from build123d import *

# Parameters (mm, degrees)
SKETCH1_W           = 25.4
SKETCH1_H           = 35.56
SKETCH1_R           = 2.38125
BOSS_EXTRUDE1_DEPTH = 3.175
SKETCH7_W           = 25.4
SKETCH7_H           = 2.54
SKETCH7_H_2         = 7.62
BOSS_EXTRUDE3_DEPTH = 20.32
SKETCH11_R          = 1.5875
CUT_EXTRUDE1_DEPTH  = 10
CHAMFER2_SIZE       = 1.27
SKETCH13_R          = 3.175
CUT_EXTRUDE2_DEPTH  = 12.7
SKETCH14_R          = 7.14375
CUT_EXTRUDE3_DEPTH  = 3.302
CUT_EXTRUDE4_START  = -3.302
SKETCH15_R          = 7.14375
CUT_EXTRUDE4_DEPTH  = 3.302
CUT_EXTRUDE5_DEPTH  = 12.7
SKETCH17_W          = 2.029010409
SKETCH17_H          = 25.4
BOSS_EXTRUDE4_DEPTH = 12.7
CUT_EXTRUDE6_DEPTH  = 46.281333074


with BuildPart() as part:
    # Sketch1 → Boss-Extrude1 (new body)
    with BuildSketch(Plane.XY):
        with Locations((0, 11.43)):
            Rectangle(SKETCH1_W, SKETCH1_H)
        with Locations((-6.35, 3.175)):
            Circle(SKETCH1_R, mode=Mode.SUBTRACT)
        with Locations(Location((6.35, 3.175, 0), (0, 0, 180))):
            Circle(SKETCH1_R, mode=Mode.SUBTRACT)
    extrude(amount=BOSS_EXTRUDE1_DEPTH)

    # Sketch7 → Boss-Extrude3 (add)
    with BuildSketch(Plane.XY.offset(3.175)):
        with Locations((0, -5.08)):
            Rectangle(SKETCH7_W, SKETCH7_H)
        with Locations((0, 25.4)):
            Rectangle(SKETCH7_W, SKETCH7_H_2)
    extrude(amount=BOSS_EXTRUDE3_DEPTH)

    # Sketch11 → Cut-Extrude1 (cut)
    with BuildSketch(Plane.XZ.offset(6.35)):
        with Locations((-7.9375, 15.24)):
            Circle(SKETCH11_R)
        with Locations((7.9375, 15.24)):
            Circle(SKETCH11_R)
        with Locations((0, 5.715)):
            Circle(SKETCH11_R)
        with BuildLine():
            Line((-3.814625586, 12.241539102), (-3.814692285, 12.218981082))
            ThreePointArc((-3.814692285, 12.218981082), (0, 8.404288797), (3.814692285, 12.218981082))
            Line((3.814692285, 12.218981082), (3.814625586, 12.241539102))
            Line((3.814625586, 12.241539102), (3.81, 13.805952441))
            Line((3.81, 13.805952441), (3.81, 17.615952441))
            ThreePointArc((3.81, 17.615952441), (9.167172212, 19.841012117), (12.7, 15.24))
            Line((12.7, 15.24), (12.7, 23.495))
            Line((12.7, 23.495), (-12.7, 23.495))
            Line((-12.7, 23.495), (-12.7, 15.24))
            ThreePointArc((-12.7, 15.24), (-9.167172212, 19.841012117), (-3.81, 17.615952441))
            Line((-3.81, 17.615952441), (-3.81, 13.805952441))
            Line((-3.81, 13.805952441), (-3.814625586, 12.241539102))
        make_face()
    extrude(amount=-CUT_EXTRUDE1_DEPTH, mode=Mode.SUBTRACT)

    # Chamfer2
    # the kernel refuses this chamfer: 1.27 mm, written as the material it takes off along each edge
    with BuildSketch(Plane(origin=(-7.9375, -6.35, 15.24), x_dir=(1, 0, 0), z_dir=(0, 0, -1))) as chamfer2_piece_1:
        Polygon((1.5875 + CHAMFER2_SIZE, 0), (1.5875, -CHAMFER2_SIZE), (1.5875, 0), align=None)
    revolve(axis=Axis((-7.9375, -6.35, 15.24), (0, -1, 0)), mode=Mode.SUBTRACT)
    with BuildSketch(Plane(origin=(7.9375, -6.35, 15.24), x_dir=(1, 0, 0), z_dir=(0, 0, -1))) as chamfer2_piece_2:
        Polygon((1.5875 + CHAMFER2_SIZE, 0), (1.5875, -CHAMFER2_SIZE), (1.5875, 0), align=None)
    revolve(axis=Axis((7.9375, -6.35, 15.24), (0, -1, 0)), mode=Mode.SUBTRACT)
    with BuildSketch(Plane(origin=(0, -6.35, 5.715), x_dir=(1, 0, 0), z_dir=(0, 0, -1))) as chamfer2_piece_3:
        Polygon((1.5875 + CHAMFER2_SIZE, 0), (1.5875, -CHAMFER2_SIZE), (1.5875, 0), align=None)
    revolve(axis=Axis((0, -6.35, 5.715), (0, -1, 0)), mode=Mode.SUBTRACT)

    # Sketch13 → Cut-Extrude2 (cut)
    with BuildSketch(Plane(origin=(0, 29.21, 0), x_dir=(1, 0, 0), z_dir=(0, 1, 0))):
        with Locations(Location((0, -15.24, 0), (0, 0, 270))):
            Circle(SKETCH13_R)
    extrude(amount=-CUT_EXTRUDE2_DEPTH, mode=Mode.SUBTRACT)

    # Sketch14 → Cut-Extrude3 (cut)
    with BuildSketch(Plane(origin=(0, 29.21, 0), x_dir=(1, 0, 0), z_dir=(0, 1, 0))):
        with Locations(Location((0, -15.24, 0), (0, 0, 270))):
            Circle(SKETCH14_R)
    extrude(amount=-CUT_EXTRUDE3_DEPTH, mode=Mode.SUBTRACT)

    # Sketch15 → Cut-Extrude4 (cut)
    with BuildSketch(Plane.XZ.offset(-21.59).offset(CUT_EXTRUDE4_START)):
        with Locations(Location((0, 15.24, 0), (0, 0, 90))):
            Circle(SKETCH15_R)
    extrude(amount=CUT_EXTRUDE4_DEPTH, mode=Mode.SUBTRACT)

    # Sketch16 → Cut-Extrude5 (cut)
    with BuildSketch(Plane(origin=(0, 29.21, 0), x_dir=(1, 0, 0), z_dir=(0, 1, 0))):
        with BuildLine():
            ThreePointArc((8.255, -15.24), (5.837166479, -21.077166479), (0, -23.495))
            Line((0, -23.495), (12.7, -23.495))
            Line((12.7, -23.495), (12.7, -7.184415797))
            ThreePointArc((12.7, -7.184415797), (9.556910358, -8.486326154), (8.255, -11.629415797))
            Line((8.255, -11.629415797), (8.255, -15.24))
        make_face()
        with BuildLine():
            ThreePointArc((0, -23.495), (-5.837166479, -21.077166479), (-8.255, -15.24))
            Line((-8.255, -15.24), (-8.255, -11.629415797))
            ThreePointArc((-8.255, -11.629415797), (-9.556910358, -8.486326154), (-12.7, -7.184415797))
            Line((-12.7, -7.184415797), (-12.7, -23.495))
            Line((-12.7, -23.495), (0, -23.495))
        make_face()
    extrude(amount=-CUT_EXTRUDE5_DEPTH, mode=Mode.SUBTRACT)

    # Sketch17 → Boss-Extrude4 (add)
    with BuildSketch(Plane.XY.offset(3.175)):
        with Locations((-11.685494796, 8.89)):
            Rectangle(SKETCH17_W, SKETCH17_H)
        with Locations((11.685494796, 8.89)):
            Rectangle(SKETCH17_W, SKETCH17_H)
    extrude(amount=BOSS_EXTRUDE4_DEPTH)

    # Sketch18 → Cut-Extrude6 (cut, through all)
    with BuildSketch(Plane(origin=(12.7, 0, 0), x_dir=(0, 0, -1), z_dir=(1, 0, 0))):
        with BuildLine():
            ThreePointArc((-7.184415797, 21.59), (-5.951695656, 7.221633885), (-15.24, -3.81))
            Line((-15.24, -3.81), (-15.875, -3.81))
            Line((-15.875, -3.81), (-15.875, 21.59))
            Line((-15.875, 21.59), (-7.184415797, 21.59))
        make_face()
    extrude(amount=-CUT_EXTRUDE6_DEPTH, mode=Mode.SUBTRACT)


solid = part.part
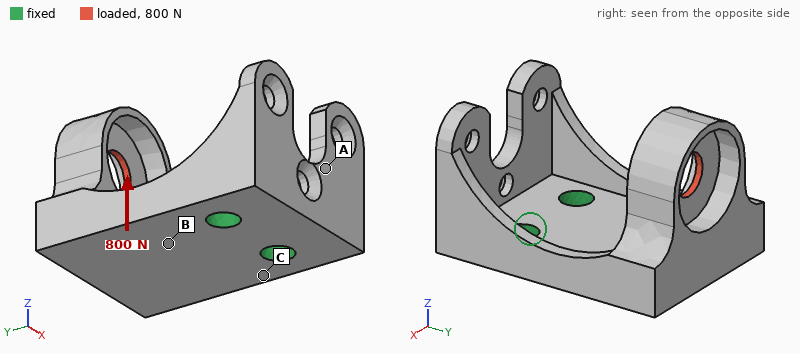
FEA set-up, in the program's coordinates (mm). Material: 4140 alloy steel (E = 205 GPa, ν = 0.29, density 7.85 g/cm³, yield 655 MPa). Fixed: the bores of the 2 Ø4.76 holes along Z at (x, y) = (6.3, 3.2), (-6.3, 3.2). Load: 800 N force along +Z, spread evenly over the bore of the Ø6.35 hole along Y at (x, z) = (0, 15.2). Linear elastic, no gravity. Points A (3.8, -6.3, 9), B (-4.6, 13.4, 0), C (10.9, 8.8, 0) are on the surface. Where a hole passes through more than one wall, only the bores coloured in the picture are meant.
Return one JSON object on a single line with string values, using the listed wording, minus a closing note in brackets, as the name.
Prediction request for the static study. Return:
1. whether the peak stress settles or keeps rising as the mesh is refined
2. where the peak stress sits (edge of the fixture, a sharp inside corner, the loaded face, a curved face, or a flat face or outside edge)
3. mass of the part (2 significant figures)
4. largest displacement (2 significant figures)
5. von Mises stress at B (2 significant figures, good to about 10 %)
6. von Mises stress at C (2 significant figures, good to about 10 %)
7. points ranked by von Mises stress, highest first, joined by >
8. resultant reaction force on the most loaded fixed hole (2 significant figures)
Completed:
{"whether the peak stress settles or keeps rising as the mesh is refined": "keeps rising", "where the peak stress sits": "edge of the fixture", "mass of the part": "43 g", "largest displacement": "0.20 mm", "von Mises stress at B": "130 MPa", "von Mises stress at C": "190 MPa", "points ranked by von Mises stress, highest first, joined by >": "C > B > A", "resultant reaction force on the most loaded fixed hole": "400 N"}
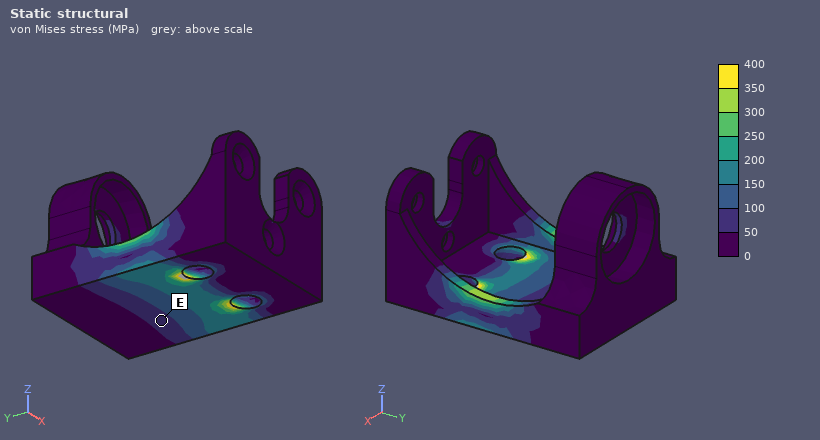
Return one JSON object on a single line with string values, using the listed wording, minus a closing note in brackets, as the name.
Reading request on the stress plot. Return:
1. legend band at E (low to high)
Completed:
{"legend band at E": "50 to 100 MPa"}
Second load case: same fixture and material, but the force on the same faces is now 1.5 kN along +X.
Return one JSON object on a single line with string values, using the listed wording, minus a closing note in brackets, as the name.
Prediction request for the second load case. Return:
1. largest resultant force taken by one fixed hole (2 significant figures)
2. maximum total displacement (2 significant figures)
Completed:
{"largest resultant force taken by one fixed hole": "2.4 kN", "maximum total displacement": "0.17 mm"}
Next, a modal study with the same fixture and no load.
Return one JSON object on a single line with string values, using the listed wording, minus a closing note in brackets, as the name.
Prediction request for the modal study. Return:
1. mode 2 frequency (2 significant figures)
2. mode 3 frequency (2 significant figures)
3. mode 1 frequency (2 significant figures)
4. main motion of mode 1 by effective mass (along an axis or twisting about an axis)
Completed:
{"mode 2 frequency": "5900 Hz", "mode 3 frequency": "10 kHz", "mode 1 frequency": "2800 Hz", "main motion of mode 1 by effective mass": "along Z"}
